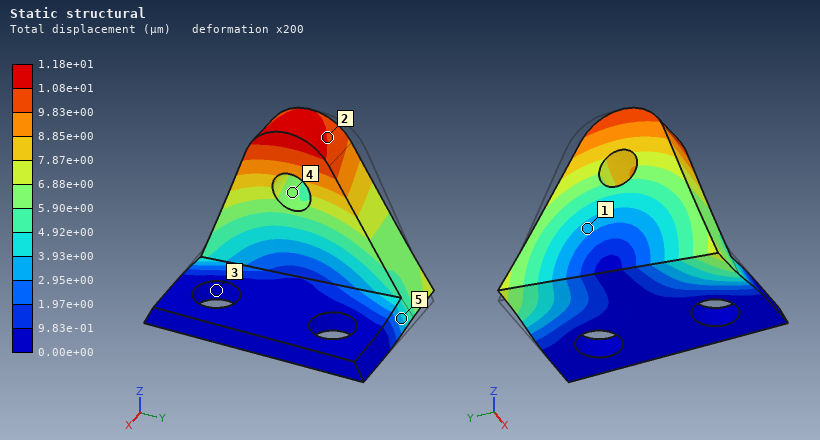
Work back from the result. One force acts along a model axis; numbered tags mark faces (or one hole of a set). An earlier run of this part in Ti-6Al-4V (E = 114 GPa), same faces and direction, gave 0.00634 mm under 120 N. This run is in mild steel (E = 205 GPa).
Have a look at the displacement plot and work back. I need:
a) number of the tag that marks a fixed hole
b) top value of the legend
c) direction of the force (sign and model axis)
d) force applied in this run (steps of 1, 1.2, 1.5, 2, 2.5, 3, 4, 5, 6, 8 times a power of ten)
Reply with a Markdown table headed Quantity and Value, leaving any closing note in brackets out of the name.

| Quantity | Value |
|---|---|
| number of the tag that marks a fixed hole | 3 |
| top value of the legend | 1.18e+01 µm |
| direction of the force | -Y |
| force applied in this run | 400 N |
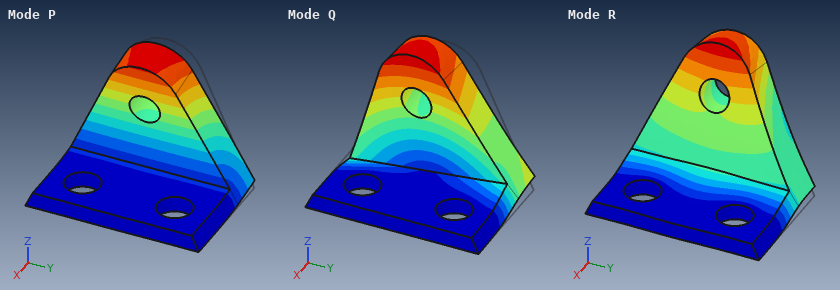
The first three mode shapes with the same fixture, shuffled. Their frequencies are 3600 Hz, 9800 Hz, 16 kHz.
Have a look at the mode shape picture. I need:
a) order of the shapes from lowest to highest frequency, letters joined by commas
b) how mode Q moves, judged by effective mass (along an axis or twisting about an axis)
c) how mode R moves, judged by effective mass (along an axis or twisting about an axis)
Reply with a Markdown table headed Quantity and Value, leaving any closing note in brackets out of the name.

| Quantity | Value |
|---|---|
| order of the shapes from lowest to highest frequency, letters joined by commas | P, Q, R |
| how mode Q moves, judged by effective mass | along Y |
| how mode R moves, judged by effective mass | along Z |
